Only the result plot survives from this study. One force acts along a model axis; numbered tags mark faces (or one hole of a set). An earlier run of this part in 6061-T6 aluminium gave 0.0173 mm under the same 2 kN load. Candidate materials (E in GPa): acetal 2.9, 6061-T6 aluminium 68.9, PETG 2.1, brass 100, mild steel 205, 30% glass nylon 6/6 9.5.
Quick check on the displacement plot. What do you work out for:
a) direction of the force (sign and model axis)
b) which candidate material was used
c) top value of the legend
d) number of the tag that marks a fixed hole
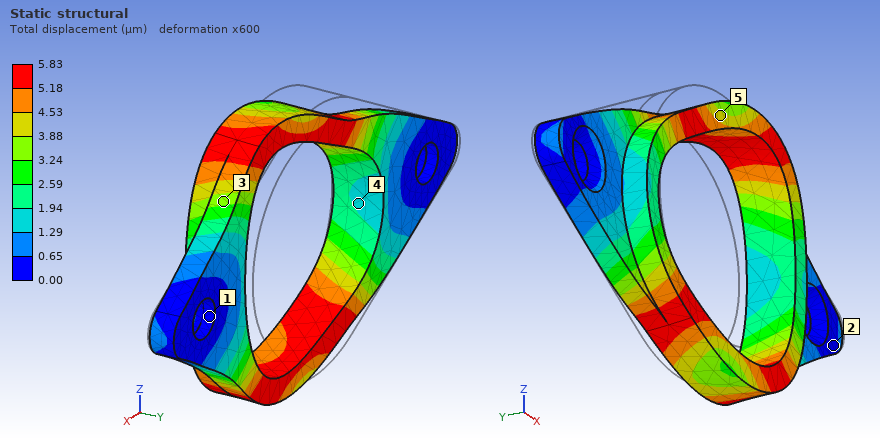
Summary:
+X
mild steel
5.83 µm
1
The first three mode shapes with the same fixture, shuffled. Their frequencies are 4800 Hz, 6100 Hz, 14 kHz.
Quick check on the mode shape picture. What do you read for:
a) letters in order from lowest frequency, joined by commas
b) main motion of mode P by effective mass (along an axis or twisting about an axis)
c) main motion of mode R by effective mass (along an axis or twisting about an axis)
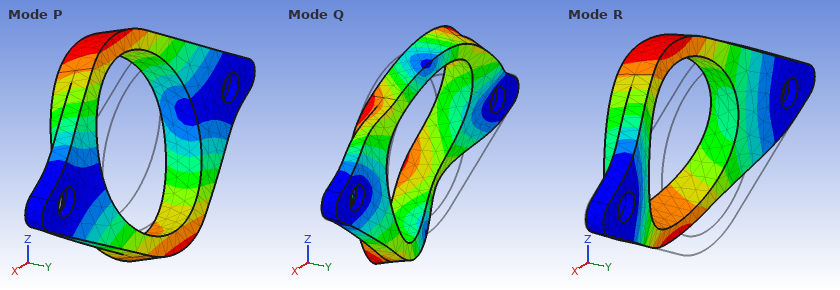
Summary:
P, R, Q
twisting about X
along Y
